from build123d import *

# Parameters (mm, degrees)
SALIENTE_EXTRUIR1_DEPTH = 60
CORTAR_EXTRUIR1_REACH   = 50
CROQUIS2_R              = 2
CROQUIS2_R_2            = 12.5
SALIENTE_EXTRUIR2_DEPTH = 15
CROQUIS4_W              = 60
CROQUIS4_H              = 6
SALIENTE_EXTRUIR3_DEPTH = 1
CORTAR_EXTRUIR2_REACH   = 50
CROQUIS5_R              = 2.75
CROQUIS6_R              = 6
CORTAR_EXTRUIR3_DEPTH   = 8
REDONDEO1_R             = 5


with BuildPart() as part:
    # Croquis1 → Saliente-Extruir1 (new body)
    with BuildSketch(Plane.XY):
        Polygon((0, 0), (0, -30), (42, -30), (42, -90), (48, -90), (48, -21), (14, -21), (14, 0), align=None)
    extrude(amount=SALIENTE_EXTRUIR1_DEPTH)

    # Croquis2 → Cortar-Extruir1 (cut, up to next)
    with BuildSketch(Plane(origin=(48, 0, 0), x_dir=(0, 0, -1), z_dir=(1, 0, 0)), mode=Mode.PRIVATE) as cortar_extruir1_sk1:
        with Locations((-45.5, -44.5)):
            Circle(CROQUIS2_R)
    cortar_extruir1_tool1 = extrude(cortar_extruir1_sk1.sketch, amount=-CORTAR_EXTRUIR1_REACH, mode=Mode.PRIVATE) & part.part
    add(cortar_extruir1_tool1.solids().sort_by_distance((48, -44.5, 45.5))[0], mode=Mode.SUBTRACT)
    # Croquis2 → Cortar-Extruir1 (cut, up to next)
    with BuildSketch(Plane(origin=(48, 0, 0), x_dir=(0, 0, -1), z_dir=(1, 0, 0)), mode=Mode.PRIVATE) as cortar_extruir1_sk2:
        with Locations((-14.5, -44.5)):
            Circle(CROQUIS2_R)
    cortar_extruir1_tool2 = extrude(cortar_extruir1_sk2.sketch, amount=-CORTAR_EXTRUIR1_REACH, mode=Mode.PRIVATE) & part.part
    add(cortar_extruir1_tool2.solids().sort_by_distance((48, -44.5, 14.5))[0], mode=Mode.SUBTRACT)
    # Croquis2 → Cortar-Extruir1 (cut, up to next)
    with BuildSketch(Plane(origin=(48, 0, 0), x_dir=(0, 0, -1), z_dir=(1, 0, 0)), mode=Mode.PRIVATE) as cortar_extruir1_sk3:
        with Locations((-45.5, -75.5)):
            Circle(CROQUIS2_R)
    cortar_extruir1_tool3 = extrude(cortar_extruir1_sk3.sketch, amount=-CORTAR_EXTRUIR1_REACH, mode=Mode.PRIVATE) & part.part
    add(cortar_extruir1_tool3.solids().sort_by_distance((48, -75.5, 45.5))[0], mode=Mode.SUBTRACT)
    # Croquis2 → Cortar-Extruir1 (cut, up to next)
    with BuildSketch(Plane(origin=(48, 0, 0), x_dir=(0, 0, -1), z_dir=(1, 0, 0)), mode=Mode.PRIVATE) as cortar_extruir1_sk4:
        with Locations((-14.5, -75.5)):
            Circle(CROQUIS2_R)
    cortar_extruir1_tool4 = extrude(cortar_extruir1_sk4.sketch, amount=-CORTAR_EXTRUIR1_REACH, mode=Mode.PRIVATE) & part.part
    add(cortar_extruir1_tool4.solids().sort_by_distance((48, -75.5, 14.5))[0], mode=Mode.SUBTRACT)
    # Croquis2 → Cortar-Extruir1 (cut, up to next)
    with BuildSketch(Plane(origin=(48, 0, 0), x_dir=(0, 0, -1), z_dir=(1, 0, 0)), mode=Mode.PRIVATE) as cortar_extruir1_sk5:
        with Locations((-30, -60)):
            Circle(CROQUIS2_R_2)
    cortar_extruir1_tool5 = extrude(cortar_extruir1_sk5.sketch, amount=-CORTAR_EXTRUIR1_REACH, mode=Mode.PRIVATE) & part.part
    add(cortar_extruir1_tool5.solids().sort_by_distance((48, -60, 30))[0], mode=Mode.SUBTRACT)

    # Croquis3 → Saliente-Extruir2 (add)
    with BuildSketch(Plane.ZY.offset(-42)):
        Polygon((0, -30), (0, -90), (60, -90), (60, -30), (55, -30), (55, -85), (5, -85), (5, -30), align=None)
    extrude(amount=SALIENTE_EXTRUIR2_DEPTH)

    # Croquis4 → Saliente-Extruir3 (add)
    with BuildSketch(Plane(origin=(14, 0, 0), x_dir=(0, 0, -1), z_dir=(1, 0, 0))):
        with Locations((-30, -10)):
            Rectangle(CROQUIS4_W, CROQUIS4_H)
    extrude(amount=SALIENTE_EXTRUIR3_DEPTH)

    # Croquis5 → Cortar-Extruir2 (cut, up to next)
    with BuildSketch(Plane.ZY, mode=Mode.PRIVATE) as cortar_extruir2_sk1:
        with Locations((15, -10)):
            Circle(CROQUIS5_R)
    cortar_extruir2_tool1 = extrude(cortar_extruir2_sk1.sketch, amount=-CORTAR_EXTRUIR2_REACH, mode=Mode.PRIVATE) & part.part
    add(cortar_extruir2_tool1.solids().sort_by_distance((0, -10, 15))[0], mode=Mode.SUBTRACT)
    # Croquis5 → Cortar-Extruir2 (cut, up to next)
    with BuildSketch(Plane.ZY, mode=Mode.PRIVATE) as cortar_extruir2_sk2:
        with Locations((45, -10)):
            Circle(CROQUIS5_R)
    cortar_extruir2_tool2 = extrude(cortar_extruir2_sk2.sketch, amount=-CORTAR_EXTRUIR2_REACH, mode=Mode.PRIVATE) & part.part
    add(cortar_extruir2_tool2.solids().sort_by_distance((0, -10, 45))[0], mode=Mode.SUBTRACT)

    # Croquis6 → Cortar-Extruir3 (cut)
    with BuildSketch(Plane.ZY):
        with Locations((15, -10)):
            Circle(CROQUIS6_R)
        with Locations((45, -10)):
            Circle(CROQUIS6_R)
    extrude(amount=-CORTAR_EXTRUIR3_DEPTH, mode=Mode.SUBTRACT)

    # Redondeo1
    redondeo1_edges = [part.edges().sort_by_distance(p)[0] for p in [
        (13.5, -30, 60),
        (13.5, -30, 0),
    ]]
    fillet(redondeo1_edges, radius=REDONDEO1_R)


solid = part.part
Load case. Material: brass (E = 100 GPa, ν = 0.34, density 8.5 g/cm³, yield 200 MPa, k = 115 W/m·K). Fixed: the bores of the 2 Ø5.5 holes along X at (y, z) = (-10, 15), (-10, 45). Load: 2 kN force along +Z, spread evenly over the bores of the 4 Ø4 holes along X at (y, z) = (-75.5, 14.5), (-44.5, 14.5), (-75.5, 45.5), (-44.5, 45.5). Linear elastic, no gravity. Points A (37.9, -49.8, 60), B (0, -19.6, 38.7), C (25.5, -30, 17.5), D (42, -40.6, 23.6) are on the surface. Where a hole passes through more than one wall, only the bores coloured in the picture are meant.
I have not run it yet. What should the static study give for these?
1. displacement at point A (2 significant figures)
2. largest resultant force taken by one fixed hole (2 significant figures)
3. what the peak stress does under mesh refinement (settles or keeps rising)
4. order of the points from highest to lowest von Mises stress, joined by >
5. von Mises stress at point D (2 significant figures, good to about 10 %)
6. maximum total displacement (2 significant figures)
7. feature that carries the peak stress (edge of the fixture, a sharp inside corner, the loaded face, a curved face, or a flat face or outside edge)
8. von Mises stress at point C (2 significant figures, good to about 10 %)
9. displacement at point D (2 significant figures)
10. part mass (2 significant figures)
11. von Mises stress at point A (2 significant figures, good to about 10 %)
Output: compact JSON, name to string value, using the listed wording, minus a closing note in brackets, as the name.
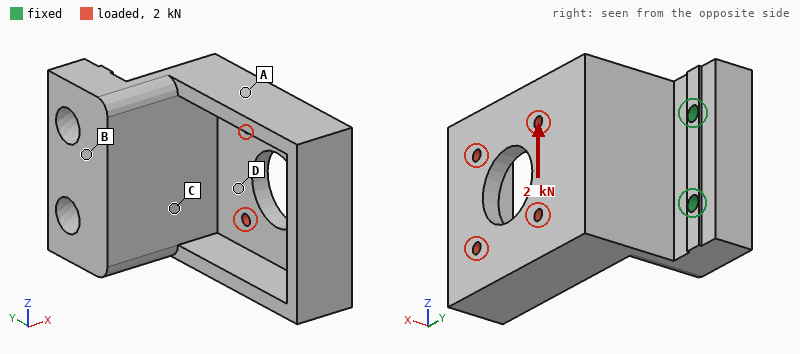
{"displacement at point A": "0.094 mm", "largest resultant force taken by one fixed hole": "3.7 kN", "what the peak stress does under mesh refinement": "keeps rising", "order of the points from highest to lowest von Mises stress, joined by >": "C > D > A > B", "von Mises stress at point D": "30 MPa", "maximum total displacement": "0.21 mm", "feature that carries the peak stress": "edge of the fixture", "von Mises stress at point C": "42 MPa", "displacement at point D": "0.053 mm", "part mass": "620 g", "von Mises stress at point A": "18 MPa"}
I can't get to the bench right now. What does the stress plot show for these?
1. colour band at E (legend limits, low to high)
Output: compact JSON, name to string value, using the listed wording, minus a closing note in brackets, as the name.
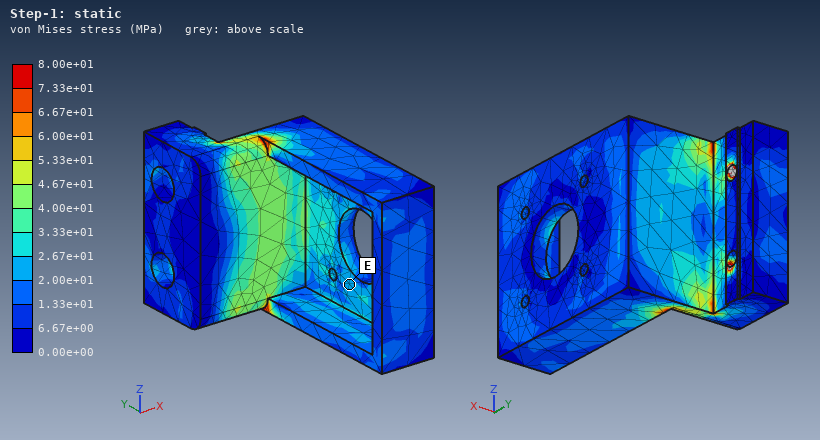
{"colour band at E": "2.00e+01 to 2.67e+01 MPa"}
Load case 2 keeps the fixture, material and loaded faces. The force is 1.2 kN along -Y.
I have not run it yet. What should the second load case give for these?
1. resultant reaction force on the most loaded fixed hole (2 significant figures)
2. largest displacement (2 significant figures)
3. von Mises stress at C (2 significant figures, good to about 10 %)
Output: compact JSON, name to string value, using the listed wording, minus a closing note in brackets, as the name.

{"resultant reaction force on the most loaded fixed hole": "650 N", "largest displacement": "0.26 mm", "von Mises stress at C": "26 MPa"}
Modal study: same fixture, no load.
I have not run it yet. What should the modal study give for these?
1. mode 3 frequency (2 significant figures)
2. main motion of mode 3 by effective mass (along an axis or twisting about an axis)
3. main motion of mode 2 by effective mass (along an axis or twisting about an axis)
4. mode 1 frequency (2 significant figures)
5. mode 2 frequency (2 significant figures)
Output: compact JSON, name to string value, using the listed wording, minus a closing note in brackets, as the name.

{"mode 3 frequency": "2100 Hz", "main motion of mode 3 by effective mass": "along Z", "main motion of mode 2 by effective mass": "along Z", "mode 1 frequency": "530 Hz", "mode 2 frequency": "970 Hz"}
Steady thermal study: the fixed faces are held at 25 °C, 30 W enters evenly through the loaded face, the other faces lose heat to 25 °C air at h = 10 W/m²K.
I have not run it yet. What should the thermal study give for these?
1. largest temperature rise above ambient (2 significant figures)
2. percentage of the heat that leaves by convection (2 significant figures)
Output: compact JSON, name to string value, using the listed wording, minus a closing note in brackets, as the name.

{"largest temperature rise above ambient": "38 K", "percentage of the heat that leaves by convection": "16 %"}
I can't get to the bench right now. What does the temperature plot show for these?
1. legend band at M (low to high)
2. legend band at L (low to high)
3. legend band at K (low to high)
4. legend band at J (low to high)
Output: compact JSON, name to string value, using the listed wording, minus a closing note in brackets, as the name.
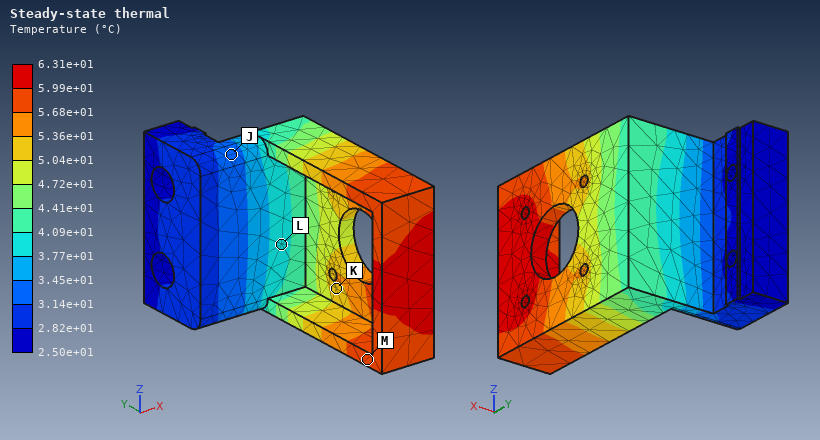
{"legend band at M": "5.68e+01 to 5.99e+01 °C", "legend band at L": "3.77e+01 to 4.09e+01 °C", "legend band at K": "5.04e+01 to 5.36e+01 °C", "legend band at J": "3.14e+01 to 3.45e+01 °C"}
